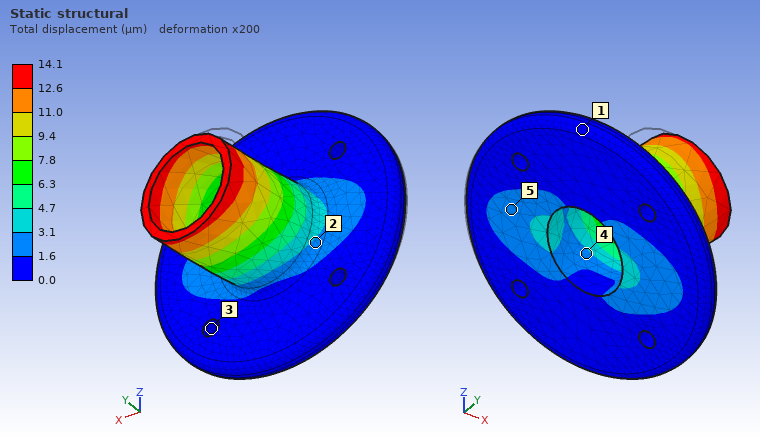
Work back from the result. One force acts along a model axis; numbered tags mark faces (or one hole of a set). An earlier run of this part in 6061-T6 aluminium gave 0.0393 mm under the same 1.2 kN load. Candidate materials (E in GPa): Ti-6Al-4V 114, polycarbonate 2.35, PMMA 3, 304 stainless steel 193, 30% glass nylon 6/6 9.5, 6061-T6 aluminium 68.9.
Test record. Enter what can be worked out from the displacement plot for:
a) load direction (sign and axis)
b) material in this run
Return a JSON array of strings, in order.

["+X", "304 stainless steel"]
